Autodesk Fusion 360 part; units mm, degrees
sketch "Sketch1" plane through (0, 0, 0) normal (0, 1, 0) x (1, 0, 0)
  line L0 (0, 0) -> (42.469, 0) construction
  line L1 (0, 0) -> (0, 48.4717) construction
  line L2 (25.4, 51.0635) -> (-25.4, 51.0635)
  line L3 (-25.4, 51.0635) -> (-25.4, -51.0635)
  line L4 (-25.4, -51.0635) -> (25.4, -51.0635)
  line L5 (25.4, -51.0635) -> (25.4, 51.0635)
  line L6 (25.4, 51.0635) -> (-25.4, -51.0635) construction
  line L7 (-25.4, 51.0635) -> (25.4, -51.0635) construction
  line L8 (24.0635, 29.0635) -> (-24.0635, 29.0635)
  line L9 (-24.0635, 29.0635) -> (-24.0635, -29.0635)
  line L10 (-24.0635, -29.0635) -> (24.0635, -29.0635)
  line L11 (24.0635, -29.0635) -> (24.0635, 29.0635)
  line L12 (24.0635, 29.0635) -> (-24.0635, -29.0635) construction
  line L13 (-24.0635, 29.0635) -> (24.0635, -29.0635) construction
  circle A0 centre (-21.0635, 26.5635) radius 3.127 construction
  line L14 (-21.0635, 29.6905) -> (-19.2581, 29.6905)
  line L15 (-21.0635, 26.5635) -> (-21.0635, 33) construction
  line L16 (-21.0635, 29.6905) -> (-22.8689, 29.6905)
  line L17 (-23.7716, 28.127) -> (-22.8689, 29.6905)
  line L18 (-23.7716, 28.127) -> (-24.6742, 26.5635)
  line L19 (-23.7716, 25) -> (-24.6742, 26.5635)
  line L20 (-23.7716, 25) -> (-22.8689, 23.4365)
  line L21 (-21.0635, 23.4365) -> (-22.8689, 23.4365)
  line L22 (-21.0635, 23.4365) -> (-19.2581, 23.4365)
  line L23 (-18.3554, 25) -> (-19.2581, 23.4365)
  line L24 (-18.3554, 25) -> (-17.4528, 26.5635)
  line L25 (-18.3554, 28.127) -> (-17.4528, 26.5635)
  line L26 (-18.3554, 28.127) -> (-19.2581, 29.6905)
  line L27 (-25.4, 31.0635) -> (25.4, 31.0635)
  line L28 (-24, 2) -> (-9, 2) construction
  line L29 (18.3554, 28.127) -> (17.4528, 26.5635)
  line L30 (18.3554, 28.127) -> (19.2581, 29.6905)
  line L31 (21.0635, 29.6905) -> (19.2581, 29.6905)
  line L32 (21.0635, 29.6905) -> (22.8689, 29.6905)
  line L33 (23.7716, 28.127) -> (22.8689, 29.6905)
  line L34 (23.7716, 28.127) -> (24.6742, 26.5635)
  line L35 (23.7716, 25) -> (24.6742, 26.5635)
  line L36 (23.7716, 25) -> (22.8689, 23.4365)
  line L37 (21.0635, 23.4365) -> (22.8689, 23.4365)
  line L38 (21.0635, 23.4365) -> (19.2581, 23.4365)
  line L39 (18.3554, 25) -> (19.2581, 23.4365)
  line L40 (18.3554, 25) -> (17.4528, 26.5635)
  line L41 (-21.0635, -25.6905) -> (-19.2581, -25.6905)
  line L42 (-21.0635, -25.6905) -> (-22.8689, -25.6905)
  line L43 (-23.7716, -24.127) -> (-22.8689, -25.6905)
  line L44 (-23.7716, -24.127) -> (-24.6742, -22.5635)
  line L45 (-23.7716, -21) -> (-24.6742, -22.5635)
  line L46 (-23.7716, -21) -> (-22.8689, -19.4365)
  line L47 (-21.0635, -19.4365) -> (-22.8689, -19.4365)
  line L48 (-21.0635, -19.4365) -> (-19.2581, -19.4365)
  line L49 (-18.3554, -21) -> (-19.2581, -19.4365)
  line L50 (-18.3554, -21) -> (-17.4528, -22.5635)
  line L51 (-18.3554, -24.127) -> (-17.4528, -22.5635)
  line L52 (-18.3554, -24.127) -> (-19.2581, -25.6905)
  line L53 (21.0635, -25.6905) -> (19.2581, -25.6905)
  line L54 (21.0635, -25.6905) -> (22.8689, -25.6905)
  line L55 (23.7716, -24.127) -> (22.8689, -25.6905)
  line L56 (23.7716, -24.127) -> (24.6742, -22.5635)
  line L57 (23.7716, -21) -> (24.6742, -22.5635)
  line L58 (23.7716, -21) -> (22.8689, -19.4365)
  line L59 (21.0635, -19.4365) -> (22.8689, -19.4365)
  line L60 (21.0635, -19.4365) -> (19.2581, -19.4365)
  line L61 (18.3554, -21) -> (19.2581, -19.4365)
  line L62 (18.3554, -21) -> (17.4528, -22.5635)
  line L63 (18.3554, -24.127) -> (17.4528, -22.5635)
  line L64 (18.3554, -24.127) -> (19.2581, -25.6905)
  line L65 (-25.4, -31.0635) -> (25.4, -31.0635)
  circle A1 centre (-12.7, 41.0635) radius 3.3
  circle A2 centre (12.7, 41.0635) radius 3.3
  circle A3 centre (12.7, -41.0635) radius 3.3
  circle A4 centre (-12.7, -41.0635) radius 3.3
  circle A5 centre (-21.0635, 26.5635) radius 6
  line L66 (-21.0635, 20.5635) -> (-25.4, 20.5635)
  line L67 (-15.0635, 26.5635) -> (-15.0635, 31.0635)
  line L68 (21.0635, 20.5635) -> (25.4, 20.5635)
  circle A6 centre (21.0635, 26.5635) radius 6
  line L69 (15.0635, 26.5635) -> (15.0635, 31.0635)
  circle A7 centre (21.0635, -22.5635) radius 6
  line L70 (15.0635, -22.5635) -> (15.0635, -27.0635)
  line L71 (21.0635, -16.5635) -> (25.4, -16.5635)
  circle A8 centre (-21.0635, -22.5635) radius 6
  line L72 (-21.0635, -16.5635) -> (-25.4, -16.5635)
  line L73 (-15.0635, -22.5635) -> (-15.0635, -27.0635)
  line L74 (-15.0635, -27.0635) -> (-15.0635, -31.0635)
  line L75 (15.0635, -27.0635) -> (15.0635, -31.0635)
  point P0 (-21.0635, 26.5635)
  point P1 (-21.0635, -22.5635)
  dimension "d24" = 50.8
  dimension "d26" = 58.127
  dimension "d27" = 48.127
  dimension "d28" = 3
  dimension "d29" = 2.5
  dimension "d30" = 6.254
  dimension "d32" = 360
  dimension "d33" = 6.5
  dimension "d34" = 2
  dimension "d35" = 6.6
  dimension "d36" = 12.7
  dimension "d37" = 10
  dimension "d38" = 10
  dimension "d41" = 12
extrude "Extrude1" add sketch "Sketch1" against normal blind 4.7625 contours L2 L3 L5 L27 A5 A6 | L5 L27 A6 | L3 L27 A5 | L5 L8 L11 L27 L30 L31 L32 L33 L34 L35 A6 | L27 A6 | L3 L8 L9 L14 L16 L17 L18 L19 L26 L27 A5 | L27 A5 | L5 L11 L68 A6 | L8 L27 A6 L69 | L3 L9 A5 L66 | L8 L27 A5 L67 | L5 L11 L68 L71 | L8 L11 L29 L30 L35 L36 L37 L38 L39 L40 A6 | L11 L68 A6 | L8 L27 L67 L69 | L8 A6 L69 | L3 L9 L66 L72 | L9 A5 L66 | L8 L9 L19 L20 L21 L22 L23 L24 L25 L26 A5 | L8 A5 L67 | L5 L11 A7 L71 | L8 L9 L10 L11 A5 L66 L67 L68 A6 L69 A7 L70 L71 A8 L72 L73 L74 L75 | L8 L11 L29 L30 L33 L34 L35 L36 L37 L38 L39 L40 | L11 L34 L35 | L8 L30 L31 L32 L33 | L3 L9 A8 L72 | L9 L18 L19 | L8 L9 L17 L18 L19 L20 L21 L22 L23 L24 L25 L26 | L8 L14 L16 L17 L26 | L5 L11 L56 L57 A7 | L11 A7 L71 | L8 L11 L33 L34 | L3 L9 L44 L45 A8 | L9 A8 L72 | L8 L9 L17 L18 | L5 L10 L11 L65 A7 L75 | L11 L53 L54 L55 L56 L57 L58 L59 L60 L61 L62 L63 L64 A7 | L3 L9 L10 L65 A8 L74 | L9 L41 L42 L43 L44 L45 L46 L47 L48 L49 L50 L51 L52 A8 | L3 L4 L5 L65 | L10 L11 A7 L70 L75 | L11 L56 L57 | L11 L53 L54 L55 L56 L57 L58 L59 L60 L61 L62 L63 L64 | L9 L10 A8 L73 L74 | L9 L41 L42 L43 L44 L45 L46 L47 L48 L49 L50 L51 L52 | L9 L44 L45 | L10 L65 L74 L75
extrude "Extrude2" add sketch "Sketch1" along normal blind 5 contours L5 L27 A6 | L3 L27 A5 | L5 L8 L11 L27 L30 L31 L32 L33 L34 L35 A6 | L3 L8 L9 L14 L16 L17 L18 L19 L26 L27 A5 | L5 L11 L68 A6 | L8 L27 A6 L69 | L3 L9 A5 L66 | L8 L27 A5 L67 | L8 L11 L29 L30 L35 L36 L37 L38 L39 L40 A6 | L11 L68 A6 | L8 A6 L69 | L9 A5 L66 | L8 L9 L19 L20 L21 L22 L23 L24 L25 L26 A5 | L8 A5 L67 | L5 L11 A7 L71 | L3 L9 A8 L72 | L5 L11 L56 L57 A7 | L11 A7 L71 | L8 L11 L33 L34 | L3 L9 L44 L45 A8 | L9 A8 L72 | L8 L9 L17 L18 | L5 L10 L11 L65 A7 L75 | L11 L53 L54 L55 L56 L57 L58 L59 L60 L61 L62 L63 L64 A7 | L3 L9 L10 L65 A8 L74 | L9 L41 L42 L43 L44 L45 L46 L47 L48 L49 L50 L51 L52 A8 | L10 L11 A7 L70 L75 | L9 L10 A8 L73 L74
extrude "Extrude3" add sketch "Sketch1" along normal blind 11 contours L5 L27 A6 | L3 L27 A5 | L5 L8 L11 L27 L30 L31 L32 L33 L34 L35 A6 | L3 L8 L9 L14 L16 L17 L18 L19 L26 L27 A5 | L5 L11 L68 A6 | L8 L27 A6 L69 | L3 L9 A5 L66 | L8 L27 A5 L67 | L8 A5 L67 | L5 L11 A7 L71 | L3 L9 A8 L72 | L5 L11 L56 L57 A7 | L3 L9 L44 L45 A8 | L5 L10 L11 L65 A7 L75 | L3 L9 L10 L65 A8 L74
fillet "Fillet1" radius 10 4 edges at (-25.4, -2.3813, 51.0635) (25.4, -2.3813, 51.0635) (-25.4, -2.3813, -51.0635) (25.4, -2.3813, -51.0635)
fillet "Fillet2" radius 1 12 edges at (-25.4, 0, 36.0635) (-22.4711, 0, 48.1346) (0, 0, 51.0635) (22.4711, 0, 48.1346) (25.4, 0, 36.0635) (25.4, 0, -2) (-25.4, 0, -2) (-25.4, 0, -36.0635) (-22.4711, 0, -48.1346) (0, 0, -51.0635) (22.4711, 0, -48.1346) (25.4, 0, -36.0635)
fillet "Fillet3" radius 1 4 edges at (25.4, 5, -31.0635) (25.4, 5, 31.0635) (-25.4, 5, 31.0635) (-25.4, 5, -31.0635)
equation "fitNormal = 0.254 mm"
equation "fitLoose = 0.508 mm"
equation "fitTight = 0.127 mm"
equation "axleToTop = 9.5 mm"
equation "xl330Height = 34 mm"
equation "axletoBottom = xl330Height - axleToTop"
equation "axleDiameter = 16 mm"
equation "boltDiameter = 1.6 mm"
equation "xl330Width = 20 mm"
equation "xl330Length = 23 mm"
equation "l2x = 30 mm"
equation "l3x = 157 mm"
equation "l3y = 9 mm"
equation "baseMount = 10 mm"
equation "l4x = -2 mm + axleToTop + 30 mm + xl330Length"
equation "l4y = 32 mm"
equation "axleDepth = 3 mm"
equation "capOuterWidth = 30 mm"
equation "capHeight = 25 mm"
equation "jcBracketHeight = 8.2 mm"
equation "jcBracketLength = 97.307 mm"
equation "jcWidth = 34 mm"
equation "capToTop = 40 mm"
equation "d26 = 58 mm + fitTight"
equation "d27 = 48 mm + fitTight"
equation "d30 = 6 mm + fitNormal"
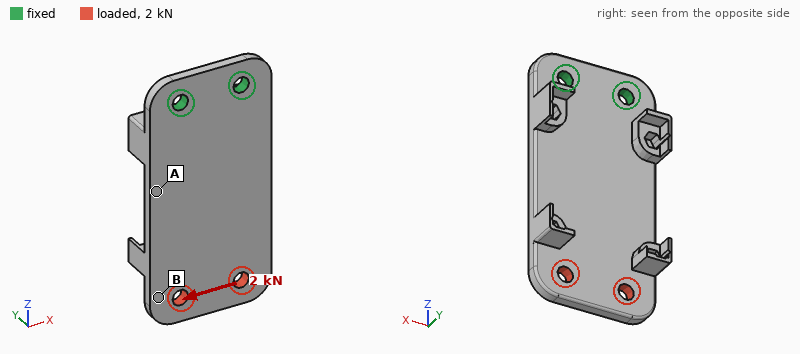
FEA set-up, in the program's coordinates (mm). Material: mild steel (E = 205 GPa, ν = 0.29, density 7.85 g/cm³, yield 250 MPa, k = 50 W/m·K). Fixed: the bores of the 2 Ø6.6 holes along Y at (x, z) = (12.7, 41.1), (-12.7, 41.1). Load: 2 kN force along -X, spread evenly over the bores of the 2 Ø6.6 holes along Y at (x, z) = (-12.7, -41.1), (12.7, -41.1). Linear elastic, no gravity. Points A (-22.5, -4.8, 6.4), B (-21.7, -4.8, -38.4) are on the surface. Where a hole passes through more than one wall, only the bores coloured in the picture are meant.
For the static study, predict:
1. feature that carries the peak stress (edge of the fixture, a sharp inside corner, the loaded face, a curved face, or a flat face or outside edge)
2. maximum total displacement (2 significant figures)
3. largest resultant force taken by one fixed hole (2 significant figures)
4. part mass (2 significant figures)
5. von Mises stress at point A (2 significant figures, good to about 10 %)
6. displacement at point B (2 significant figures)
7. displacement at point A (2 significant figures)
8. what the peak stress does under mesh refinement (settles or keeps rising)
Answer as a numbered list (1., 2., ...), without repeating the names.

1. edge of the fixture
2. 62 µm
3. 5.5 kN
4. 210 g
5. 38 MPa
6. 53 µm
7. 20 µm
8. keeps rising
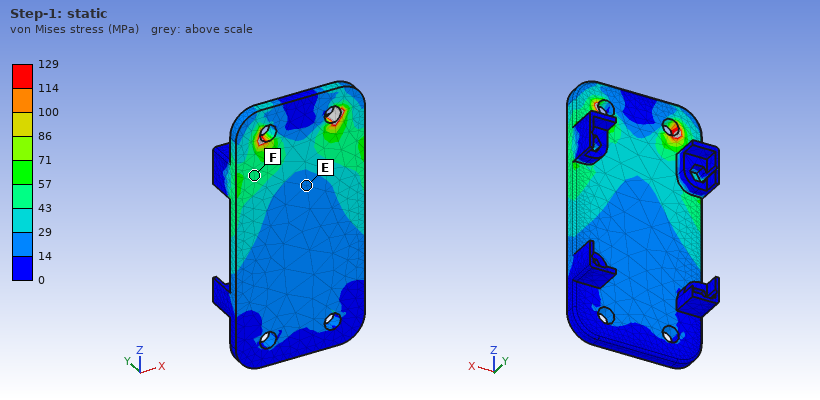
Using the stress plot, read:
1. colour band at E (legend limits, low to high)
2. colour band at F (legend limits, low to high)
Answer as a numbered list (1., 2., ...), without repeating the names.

1. 14 to 29 MPa
2. 43 to 57 MPa
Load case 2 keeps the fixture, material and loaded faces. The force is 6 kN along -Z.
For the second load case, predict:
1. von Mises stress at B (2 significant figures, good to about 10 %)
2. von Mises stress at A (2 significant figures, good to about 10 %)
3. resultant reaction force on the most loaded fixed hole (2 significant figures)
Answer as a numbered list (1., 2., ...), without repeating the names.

1. 15 MPa
2. 24 MPa
3. 3.0 kN
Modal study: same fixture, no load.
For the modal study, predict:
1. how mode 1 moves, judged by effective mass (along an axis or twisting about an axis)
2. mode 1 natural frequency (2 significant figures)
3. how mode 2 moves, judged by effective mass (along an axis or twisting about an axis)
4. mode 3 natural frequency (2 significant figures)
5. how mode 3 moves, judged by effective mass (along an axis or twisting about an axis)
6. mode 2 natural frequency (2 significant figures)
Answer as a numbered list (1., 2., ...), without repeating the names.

1. along Y
2. 510 Hz
3. twisting about Z
4. 3000 Hz
5. along Y
6. 1800 Hz
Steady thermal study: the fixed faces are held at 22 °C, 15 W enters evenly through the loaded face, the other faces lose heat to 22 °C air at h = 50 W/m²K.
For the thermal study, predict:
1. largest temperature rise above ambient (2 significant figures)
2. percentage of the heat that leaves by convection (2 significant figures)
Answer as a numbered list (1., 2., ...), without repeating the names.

1. 47 K
2. 76 %
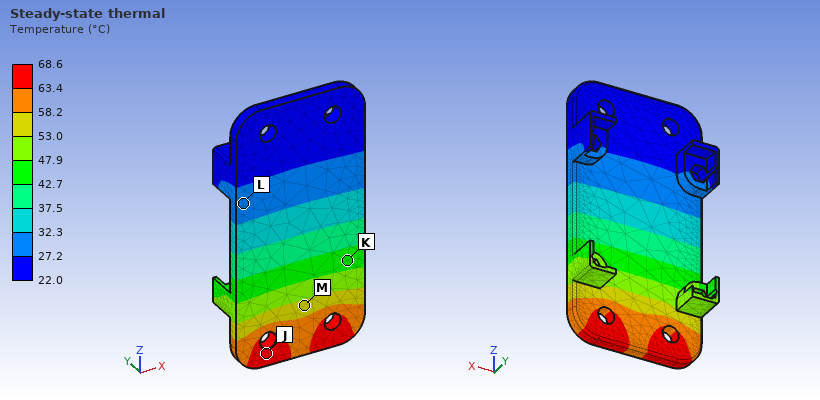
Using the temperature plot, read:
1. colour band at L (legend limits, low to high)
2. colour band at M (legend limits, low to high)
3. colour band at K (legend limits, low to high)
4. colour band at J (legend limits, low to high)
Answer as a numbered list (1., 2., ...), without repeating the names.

1. 27.2 to 32.3 °C
2. 53.0 to 58.2 °C
3. 42.7 to 47.9 °C
4. 63.4 to 68.6 °C
